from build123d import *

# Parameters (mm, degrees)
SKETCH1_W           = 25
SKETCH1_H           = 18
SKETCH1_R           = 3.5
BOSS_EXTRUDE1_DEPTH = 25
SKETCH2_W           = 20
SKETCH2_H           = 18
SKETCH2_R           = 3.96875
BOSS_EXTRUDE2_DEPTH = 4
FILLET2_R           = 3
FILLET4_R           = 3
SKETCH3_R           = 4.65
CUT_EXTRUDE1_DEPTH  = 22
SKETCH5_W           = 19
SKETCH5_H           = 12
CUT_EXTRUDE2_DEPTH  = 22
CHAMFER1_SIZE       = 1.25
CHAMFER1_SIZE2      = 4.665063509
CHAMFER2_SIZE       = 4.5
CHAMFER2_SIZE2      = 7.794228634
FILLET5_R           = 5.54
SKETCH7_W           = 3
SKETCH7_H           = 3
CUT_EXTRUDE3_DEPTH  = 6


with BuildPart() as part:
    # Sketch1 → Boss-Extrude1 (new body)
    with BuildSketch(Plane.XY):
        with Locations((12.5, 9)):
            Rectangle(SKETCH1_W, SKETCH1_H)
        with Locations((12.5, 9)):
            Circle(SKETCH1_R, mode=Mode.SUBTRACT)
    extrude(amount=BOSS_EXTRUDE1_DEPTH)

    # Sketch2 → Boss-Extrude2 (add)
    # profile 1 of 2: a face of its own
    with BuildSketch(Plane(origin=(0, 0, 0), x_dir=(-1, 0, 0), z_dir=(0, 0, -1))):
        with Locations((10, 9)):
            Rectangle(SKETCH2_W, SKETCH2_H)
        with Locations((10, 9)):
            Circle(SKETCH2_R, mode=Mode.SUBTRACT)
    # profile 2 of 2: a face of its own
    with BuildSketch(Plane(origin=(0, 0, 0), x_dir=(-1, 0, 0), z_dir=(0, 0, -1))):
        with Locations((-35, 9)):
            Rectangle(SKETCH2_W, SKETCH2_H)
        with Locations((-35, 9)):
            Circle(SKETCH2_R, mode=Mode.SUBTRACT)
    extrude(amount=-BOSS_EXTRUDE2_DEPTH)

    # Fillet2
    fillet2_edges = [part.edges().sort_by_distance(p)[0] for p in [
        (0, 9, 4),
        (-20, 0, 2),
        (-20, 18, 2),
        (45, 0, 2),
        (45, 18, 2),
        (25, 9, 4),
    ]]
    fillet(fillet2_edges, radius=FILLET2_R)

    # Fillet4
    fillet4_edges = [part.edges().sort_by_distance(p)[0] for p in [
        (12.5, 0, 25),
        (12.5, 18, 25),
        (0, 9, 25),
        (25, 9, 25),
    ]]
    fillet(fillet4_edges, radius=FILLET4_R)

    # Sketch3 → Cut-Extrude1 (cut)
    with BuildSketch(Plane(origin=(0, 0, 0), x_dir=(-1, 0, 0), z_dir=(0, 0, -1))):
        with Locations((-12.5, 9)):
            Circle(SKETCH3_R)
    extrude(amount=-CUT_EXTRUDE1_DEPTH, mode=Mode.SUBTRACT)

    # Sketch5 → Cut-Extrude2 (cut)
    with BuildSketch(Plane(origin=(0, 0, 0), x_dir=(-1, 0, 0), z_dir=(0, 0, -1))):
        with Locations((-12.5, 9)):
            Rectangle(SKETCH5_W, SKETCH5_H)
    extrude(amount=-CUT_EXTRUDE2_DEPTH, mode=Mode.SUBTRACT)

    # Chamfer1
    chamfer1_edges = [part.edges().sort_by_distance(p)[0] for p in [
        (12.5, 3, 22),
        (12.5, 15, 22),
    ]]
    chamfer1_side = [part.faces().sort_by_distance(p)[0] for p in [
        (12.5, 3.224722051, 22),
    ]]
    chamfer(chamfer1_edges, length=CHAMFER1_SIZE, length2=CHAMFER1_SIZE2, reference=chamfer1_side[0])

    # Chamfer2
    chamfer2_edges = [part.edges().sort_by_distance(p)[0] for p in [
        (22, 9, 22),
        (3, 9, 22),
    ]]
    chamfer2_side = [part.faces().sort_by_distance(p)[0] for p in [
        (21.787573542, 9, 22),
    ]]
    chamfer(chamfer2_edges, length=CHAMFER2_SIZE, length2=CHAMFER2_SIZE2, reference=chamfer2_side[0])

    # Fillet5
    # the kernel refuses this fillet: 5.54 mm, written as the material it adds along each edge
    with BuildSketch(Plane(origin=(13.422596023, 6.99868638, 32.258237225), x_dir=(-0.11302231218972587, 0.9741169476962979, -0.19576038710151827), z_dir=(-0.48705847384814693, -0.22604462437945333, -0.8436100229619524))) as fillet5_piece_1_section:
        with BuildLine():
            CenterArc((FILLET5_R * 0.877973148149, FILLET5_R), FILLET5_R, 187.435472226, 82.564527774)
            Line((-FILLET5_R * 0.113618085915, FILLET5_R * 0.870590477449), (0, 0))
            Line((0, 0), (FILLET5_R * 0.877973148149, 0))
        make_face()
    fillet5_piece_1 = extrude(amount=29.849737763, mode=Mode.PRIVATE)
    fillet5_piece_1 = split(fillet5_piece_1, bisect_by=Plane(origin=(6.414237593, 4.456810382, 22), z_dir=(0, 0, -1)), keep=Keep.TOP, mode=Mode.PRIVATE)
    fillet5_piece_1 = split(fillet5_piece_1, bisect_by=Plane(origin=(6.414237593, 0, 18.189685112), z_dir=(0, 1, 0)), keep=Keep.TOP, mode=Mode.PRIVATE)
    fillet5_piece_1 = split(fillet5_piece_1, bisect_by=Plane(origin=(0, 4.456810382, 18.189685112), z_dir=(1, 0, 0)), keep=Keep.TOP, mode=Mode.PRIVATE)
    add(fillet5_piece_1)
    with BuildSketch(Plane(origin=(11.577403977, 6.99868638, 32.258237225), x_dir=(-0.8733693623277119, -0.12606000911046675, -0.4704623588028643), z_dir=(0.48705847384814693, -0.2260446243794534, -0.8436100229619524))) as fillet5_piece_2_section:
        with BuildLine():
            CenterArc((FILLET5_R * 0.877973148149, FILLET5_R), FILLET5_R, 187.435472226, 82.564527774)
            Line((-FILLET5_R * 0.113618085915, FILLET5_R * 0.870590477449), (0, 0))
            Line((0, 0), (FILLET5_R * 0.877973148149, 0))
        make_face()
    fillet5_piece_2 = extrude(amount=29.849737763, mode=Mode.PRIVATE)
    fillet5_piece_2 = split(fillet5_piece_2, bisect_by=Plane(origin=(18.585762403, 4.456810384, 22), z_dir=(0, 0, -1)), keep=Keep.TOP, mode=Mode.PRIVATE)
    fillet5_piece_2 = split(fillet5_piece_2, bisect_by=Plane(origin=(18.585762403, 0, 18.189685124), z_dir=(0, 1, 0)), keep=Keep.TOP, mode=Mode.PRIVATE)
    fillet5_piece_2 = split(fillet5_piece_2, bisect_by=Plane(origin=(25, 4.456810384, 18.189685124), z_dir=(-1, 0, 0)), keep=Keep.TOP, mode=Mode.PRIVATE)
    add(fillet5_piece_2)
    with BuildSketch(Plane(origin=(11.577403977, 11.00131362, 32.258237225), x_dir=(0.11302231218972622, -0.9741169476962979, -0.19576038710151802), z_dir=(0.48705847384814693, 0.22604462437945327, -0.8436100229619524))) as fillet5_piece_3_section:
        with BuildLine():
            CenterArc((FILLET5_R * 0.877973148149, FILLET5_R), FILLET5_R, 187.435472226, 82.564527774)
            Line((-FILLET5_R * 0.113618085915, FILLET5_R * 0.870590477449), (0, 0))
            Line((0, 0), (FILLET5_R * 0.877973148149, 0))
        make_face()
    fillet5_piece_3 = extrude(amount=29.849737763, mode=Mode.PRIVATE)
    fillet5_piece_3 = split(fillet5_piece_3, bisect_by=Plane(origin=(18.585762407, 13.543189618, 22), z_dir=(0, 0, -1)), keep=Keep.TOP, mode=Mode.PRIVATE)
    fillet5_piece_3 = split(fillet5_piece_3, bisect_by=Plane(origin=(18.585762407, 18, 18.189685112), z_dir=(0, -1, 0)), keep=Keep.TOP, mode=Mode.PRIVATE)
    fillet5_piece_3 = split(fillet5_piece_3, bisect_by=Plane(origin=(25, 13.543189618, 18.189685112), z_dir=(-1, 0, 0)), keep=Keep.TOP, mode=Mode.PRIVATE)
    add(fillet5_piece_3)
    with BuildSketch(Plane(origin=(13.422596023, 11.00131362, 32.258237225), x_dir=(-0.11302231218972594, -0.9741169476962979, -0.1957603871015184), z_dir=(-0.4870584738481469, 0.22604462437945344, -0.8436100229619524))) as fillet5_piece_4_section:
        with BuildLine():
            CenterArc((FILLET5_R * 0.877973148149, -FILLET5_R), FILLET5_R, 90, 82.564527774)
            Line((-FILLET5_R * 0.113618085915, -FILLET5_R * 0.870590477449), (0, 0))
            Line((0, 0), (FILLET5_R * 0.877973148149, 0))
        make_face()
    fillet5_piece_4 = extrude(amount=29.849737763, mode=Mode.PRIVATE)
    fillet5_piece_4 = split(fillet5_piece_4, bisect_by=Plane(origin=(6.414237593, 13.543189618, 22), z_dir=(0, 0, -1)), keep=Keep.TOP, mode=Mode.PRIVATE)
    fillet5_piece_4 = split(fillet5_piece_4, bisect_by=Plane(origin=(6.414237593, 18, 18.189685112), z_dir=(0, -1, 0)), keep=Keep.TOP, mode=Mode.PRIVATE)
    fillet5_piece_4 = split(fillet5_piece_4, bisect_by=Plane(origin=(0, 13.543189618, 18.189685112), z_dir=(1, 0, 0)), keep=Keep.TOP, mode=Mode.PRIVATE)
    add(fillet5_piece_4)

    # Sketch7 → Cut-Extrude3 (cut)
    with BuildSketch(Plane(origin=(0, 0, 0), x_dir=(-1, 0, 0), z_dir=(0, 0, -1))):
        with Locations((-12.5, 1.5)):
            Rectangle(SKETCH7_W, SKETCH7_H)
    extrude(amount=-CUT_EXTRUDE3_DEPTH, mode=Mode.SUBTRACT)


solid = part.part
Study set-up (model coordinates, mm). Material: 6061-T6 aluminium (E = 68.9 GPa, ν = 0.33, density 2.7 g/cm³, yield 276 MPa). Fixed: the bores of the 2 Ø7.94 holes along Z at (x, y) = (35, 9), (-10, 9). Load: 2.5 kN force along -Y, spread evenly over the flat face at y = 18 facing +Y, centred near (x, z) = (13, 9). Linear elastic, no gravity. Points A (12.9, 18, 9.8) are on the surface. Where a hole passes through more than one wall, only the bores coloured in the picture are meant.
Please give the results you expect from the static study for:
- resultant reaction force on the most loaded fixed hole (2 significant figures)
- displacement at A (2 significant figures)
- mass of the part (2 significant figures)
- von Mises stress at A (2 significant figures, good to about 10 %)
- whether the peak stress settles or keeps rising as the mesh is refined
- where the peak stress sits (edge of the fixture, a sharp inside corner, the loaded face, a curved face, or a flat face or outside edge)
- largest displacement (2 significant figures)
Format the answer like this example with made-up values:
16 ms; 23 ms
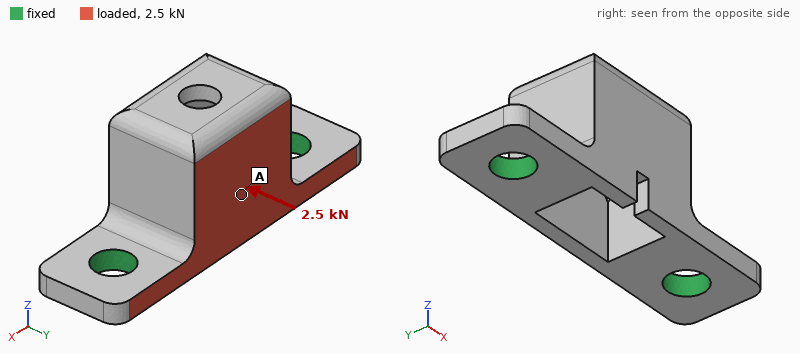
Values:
1.3 kN; 0.076 mm; 25 g; 33 MPa; keeps rising; edge of the fixture; 0.13 mm
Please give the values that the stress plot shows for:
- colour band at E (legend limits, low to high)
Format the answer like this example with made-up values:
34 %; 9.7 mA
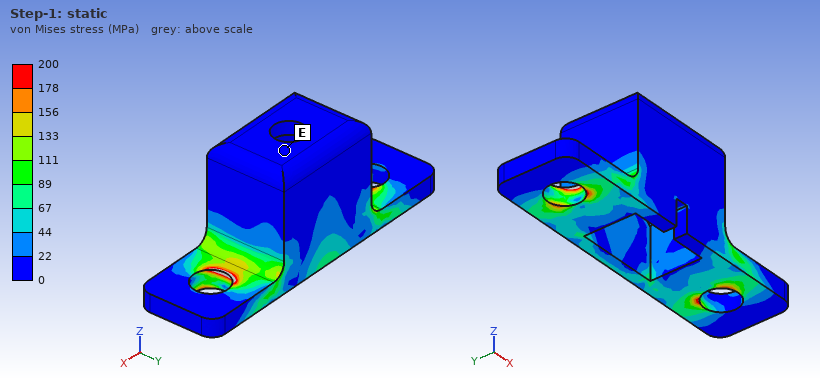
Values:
0 to 22 MPa
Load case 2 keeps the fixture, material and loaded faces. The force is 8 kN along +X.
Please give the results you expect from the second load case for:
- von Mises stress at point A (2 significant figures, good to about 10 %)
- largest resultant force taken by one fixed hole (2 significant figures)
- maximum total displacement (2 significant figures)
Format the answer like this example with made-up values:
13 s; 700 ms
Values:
92 MPa; 4.5 kN; 66 µm
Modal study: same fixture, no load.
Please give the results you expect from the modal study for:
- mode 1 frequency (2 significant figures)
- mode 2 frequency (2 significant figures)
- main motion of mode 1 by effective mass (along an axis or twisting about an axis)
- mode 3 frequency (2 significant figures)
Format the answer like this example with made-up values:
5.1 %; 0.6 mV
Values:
4600 Hz; 12 kHz; along Y; 13 kHz
